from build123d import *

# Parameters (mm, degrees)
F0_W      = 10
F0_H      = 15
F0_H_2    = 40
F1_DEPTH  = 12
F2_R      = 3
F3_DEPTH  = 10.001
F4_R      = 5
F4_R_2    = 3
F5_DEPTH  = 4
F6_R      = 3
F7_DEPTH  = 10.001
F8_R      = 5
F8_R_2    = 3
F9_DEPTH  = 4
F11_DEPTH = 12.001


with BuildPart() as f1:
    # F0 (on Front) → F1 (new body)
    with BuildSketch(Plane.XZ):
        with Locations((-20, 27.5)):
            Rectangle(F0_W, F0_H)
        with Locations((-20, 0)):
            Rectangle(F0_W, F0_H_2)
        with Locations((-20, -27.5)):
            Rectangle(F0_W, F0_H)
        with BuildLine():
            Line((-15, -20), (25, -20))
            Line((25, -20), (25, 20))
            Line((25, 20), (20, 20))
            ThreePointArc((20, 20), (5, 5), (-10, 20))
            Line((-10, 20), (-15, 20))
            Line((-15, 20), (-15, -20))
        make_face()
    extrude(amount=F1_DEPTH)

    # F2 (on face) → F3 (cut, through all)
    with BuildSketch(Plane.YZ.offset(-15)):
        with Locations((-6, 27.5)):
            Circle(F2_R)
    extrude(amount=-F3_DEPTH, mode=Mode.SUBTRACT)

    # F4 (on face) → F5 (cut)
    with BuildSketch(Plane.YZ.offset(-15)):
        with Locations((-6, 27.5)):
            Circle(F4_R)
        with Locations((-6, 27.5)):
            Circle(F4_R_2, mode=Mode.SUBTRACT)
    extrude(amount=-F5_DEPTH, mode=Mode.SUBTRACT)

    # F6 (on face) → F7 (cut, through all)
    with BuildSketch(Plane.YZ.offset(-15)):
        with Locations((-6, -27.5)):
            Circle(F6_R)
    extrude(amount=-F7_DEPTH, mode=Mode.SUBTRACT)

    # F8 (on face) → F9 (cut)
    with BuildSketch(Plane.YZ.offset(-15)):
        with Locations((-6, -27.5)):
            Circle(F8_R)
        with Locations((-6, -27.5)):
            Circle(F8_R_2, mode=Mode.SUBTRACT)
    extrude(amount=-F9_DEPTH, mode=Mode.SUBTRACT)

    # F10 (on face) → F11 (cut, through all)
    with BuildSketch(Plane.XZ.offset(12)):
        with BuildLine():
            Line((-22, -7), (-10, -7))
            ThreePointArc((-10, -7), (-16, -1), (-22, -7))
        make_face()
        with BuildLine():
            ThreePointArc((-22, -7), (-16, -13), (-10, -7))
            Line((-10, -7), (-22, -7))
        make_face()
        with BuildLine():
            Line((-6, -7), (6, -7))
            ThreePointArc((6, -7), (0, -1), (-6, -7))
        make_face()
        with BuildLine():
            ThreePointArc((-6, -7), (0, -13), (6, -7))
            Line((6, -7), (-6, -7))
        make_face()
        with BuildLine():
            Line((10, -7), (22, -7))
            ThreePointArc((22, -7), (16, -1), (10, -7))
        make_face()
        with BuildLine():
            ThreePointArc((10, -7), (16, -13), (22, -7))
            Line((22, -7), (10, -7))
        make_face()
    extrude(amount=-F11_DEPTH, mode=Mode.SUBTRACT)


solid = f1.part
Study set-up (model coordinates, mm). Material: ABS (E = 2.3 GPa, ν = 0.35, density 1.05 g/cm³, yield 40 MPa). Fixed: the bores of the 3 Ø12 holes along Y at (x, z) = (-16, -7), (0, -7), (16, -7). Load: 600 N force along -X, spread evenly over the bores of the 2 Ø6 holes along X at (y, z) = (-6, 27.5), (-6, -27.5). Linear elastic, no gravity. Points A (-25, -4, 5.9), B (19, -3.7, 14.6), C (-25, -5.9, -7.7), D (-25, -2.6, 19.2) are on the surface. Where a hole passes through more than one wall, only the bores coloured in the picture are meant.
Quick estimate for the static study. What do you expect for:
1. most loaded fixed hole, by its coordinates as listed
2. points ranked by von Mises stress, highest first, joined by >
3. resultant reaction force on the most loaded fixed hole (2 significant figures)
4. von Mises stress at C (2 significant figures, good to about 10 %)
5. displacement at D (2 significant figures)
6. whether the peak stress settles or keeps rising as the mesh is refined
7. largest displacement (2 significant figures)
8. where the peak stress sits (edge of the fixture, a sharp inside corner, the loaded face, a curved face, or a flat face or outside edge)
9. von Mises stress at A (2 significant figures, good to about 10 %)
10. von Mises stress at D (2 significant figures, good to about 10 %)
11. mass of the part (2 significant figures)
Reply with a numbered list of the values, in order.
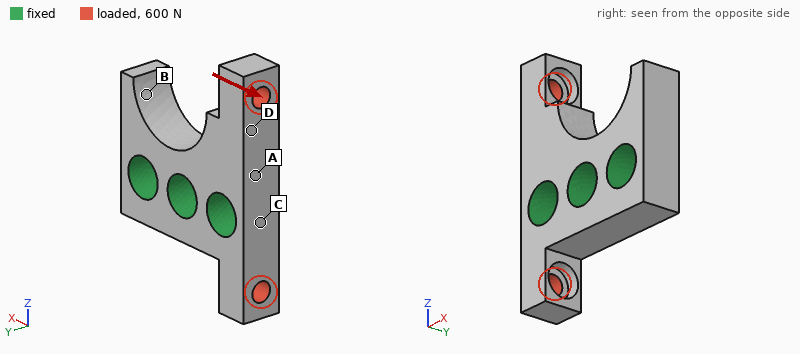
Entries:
1. (0, -7)
2. D > A > C > B
3. 500 N
4. 5.1 MPa
5. 0.14 mm
6. keeps rising
7. 0.44 mm
8. a sharp inside corner
9. 7.8 MPa
10. 12 MPa
11. 19 g
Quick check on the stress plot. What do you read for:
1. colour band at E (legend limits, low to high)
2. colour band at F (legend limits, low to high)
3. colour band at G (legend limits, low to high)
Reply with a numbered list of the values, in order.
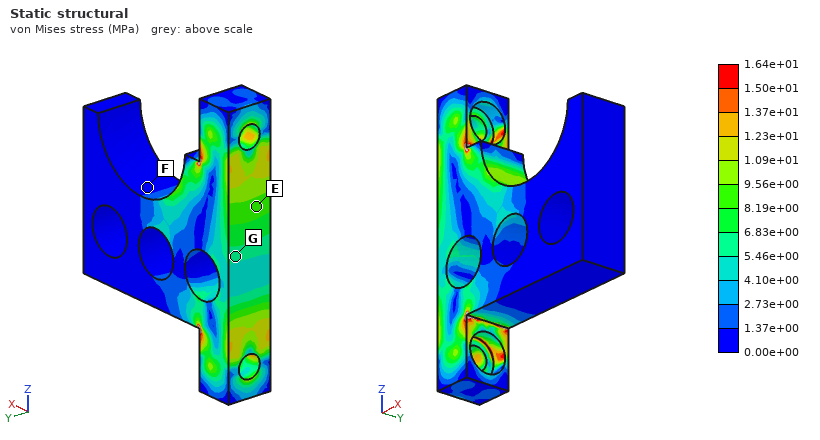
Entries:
1. 8.19e+00 to 9.56e+00 MPa
2. 0.00e+00 to 1.37e+00 MPa
3. 5.46e+00 to 6.83e+00 MPa
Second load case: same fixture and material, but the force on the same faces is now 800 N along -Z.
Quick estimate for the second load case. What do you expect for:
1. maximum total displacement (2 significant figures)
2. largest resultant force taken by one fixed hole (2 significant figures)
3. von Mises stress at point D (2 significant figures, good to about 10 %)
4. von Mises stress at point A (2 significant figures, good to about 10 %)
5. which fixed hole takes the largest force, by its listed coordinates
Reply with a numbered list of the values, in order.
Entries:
1. 0.17 mm
2. 890 N
3. 7.0 MPa
4. 4.8 MPa
5. (-16, -7)
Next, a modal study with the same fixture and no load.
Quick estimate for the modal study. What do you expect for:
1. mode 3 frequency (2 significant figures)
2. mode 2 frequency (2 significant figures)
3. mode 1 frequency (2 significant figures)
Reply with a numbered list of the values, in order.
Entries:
1. 4600 Hz
2. 3900 Hz
3. 2700 Hz
